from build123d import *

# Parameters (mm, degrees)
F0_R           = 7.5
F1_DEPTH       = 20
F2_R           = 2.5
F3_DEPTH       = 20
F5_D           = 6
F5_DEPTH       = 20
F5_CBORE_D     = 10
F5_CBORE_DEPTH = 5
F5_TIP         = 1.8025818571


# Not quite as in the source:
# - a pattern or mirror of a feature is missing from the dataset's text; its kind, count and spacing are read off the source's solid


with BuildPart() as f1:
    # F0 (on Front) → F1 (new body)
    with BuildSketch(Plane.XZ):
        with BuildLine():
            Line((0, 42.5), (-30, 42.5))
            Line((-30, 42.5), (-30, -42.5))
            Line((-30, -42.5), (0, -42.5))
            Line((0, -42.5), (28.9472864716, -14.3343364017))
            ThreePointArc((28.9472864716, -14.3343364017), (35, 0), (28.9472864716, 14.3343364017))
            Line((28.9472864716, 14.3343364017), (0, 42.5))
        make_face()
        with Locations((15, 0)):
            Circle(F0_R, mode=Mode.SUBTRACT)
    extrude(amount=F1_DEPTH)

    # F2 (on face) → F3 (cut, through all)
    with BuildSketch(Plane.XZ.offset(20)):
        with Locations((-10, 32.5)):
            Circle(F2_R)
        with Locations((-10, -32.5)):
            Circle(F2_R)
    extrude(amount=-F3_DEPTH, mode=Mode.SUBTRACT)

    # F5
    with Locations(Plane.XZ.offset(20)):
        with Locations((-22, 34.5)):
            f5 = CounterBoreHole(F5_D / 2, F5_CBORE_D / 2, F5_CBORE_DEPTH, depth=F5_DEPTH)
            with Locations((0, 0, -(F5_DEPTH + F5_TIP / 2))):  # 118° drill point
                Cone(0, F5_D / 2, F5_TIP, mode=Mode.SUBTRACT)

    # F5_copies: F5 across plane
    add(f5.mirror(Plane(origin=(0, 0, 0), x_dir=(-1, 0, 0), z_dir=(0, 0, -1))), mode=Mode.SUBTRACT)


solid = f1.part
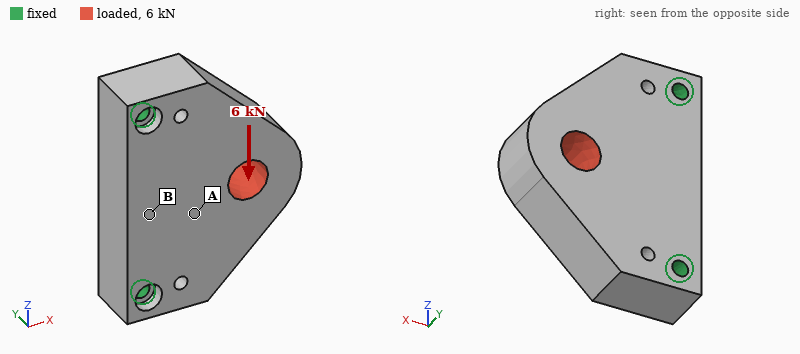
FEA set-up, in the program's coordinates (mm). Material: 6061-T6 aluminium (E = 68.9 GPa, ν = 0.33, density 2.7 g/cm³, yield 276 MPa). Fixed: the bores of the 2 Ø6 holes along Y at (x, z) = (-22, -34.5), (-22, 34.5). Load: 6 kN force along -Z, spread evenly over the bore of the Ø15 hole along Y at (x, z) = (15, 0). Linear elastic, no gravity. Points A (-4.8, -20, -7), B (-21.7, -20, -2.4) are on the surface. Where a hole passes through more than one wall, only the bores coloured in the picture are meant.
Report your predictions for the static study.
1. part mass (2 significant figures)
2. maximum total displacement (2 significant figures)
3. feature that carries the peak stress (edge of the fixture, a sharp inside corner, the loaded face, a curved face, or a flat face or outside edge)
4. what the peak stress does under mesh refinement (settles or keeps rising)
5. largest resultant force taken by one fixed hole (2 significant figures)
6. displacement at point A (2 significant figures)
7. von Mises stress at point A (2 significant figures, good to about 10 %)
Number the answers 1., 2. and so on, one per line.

1. 220 g
2. 13 µm
3. edge of the fixture
4. keeps rising
5. 4.3 kN
6. 4.6 µm
7. 7.3 MPa
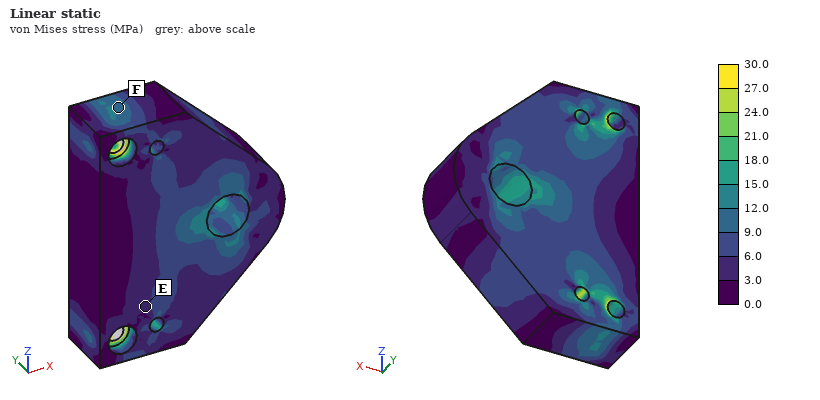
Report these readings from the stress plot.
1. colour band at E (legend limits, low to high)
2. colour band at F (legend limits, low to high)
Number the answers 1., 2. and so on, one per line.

1. 3.0 to 6.0 MPa
2. 9.0 to 12.0 MPa
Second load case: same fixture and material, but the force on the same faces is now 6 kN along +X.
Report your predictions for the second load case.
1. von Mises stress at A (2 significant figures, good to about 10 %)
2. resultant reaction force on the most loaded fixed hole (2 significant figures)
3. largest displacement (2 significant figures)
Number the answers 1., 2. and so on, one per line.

1. 4.7 MPa
2. 3.3 kN
3. 11 µm
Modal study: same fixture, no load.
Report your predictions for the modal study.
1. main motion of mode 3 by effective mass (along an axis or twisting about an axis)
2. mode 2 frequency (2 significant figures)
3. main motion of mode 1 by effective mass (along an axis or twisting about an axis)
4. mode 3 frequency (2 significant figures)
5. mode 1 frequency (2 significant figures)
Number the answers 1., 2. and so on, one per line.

1. along Z
2. 12 kHz
3. along Y
4. 13 kHz
5. 3800 Hz
